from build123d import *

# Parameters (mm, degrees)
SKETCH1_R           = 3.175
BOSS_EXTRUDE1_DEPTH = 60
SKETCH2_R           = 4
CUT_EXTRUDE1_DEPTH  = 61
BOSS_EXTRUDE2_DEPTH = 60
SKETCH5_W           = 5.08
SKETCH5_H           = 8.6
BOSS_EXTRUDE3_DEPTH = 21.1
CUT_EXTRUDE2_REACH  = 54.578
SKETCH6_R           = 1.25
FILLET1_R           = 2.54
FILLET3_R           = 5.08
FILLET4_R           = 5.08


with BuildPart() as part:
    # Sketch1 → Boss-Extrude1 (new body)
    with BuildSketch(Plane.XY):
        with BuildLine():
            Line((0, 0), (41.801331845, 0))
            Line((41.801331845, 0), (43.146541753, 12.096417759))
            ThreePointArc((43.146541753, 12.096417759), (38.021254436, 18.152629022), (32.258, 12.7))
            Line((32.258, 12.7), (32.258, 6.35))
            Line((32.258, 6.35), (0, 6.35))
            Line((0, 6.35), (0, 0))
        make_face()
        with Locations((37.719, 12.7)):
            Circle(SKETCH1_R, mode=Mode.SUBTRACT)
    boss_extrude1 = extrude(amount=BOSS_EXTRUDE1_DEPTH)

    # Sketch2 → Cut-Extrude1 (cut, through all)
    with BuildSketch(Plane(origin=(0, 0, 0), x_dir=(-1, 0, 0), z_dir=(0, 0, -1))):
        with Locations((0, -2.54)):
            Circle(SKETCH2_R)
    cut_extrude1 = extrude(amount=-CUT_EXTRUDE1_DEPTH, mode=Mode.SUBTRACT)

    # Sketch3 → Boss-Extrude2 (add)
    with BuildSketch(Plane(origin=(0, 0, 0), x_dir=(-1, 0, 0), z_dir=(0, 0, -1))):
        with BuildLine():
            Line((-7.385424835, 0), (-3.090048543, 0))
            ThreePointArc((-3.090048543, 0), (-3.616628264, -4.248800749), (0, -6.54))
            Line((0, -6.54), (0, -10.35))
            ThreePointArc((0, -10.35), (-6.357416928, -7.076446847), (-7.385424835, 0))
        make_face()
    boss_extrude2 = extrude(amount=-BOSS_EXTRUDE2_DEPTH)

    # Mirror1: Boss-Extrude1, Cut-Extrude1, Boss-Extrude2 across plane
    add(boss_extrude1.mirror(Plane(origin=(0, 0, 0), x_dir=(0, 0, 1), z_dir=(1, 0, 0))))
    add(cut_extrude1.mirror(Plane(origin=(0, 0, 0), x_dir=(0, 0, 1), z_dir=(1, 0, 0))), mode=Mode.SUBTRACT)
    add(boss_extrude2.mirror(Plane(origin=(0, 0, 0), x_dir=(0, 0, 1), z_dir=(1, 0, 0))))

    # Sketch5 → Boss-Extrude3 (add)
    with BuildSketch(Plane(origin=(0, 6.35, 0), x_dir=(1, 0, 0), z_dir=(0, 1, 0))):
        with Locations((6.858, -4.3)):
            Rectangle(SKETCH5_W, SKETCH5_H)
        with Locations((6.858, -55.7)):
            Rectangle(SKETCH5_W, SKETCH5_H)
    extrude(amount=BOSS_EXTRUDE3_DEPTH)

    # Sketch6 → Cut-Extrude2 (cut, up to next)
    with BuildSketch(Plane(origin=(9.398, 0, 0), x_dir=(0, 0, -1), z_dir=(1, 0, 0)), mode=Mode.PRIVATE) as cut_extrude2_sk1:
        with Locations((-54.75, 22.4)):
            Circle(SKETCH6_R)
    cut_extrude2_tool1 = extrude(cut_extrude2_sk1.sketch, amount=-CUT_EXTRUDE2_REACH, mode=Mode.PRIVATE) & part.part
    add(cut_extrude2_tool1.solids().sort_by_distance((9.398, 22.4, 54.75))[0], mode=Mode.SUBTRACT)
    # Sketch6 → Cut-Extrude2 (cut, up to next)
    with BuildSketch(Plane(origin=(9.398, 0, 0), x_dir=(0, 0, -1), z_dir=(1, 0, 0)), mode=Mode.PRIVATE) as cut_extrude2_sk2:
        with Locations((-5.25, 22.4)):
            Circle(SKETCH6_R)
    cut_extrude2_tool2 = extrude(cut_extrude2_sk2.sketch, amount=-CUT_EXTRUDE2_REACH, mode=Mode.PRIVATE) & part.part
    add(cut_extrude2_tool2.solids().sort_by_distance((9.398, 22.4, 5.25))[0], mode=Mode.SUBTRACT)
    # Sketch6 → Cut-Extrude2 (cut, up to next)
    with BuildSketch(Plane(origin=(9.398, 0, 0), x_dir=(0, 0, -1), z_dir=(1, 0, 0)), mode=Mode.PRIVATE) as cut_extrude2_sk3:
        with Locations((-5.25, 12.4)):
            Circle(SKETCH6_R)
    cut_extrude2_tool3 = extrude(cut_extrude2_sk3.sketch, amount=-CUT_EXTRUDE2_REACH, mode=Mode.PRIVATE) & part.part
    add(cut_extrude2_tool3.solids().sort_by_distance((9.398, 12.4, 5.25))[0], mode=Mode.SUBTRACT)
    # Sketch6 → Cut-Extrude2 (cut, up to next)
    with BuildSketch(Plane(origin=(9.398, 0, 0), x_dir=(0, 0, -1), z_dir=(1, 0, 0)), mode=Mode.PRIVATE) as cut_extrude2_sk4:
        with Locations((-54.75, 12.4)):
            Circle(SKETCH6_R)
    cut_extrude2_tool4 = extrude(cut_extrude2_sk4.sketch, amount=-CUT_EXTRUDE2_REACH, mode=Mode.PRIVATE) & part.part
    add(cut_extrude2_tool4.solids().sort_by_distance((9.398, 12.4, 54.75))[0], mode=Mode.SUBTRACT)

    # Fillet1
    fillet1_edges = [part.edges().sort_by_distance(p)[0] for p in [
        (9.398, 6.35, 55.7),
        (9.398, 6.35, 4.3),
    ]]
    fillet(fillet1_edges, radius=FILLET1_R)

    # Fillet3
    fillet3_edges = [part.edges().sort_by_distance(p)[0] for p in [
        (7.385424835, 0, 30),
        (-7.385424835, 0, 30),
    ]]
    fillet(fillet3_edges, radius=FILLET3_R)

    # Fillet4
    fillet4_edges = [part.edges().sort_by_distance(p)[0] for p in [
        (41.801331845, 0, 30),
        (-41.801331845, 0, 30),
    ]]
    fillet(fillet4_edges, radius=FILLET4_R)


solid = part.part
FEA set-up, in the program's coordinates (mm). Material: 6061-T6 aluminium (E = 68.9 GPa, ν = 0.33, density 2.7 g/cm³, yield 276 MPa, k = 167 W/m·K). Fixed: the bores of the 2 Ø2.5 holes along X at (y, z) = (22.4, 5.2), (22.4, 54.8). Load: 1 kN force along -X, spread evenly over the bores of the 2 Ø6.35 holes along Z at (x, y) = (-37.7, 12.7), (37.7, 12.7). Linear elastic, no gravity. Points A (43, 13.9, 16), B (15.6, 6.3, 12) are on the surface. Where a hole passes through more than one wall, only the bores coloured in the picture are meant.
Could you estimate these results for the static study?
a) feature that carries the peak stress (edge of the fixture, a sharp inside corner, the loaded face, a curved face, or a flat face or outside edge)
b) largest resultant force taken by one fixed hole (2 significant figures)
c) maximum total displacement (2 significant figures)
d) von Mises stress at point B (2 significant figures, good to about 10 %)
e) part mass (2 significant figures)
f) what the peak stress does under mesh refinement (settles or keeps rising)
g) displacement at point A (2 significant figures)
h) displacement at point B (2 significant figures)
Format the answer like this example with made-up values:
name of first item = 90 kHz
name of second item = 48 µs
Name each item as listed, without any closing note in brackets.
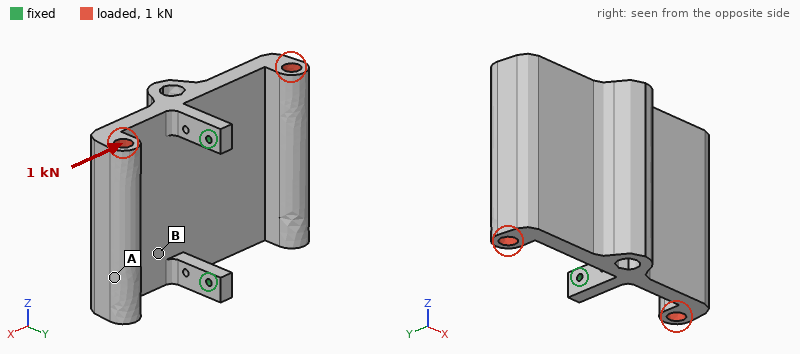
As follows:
feature that carries the peak stress = edge of the fixture
largest resultant force taken by one fixed hole = 500 N
maximum total displacement = 78 µm
von Mises stress at point B = 13 MPa
part mass = 130 g
what the peak stress does under mesh refinement = keeps rising
displacement at point A = 63 µm
displacement at point B = 56 µm
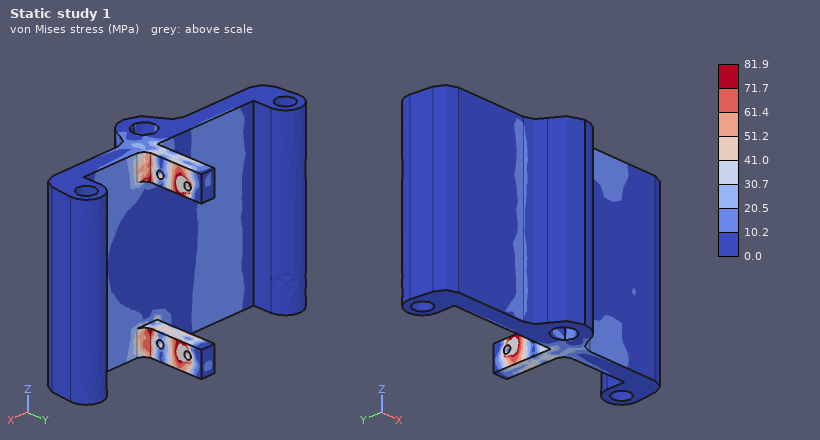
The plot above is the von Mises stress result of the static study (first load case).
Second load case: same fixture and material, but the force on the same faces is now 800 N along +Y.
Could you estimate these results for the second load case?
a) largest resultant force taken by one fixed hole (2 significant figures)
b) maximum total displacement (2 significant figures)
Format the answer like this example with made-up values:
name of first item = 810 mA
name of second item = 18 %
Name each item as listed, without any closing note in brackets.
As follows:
largest resultant force taken by one fixed hole = 400 N
maximum total displacement = 0.49 mm
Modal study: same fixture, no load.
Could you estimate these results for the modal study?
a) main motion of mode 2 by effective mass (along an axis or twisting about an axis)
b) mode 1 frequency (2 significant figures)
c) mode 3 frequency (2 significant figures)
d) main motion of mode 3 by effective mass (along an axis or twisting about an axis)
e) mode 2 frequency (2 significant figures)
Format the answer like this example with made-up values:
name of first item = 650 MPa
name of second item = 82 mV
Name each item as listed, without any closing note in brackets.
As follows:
main motion of mode 2 by effective mass = along Z
mode 1 frequency = 400 Hz
mode 3 frequency = 2100 Hz
main motion of mode 3 by effective mass = along X
mode 2 frequency = 1600 Hz
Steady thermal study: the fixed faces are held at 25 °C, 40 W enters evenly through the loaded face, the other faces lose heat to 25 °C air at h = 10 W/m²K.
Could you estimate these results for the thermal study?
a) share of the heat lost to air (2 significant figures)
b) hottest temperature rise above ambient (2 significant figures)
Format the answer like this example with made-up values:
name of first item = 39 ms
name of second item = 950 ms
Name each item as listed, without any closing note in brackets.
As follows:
share of the heat lost to air = 21 %
hottest temperature rise above ambient = 55 K
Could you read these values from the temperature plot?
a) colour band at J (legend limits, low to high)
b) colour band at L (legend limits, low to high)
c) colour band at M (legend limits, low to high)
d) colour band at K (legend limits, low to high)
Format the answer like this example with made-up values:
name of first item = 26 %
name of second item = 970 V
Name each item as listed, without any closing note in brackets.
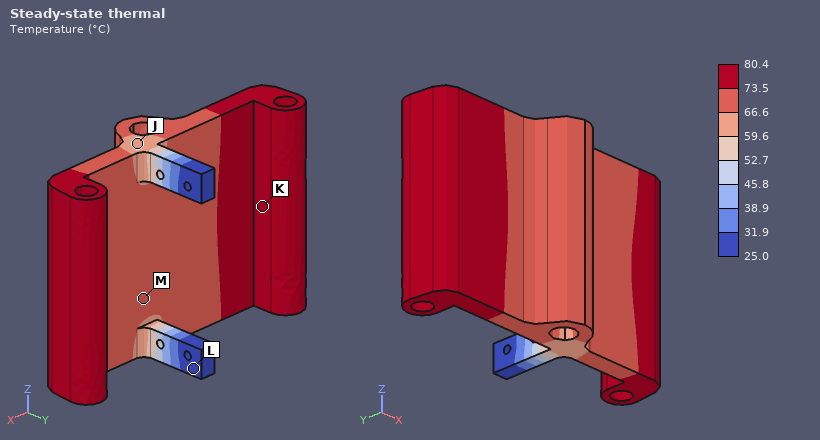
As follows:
colour band at J = 59.6 to 66.6 °C
colour band at L = 25.0 to 31.9 °C
colour band at M = 66.6 to 73.5 °C
colour band at K = 73.5 to 80.4 °C
